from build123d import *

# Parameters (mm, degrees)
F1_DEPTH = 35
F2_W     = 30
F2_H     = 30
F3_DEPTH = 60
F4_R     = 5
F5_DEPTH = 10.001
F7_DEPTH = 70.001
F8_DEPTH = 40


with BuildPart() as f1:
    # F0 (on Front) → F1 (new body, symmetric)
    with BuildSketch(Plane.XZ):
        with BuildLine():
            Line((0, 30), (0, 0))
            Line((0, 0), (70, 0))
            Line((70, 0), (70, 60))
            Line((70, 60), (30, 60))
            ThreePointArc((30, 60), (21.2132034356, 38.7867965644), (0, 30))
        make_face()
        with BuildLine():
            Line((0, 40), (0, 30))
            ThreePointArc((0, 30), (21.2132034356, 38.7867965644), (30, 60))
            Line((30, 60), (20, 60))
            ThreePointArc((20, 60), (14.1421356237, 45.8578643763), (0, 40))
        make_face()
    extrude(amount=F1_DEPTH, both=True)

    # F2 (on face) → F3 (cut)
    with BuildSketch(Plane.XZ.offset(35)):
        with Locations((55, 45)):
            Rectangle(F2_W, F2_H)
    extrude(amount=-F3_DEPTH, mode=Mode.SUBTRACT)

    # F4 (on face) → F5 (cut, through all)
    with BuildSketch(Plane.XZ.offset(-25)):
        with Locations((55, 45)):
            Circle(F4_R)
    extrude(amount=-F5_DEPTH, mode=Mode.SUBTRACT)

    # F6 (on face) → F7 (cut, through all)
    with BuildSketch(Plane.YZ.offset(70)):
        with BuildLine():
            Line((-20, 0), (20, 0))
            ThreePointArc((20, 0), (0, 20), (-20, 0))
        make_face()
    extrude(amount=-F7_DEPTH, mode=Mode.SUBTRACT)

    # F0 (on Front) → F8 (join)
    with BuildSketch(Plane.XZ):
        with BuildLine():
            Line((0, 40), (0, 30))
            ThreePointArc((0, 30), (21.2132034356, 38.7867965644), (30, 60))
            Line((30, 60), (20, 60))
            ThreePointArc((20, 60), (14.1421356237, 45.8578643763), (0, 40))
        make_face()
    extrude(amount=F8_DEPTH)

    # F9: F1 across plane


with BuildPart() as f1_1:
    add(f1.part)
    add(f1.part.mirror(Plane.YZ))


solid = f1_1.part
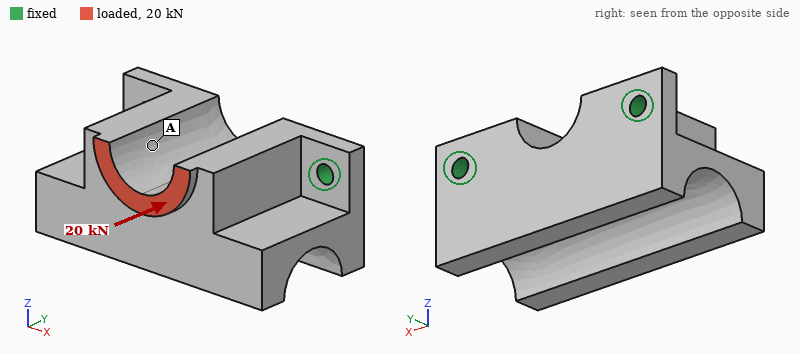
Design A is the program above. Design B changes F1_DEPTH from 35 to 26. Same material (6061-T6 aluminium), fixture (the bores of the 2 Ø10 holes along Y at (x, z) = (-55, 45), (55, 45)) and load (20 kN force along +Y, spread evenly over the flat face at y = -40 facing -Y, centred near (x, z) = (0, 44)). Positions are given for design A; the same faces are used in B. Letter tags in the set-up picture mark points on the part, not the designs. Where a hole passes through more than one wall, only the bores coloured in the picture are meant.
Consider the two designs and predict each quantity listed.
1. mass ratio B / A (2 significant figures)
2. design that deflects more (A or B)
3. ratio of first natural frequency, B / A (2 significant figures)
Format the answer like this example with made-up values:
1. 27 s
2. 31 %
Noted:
1. 0.67
2. B
3. 0.092
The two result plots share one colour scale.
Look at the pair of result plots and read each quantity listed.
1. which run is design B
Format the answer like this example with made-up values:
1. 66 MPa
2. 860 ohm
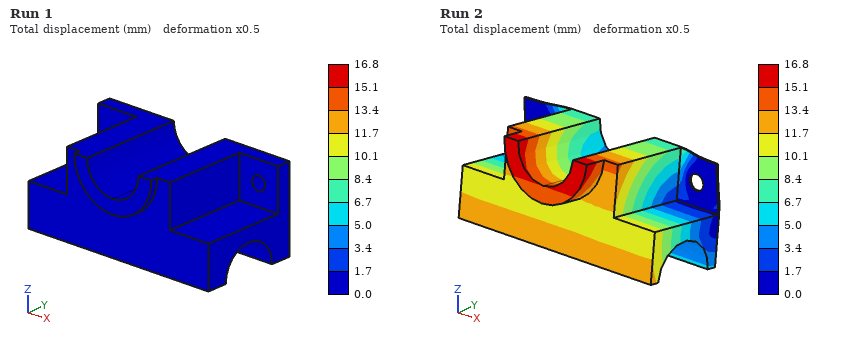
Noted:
1. Run 2
